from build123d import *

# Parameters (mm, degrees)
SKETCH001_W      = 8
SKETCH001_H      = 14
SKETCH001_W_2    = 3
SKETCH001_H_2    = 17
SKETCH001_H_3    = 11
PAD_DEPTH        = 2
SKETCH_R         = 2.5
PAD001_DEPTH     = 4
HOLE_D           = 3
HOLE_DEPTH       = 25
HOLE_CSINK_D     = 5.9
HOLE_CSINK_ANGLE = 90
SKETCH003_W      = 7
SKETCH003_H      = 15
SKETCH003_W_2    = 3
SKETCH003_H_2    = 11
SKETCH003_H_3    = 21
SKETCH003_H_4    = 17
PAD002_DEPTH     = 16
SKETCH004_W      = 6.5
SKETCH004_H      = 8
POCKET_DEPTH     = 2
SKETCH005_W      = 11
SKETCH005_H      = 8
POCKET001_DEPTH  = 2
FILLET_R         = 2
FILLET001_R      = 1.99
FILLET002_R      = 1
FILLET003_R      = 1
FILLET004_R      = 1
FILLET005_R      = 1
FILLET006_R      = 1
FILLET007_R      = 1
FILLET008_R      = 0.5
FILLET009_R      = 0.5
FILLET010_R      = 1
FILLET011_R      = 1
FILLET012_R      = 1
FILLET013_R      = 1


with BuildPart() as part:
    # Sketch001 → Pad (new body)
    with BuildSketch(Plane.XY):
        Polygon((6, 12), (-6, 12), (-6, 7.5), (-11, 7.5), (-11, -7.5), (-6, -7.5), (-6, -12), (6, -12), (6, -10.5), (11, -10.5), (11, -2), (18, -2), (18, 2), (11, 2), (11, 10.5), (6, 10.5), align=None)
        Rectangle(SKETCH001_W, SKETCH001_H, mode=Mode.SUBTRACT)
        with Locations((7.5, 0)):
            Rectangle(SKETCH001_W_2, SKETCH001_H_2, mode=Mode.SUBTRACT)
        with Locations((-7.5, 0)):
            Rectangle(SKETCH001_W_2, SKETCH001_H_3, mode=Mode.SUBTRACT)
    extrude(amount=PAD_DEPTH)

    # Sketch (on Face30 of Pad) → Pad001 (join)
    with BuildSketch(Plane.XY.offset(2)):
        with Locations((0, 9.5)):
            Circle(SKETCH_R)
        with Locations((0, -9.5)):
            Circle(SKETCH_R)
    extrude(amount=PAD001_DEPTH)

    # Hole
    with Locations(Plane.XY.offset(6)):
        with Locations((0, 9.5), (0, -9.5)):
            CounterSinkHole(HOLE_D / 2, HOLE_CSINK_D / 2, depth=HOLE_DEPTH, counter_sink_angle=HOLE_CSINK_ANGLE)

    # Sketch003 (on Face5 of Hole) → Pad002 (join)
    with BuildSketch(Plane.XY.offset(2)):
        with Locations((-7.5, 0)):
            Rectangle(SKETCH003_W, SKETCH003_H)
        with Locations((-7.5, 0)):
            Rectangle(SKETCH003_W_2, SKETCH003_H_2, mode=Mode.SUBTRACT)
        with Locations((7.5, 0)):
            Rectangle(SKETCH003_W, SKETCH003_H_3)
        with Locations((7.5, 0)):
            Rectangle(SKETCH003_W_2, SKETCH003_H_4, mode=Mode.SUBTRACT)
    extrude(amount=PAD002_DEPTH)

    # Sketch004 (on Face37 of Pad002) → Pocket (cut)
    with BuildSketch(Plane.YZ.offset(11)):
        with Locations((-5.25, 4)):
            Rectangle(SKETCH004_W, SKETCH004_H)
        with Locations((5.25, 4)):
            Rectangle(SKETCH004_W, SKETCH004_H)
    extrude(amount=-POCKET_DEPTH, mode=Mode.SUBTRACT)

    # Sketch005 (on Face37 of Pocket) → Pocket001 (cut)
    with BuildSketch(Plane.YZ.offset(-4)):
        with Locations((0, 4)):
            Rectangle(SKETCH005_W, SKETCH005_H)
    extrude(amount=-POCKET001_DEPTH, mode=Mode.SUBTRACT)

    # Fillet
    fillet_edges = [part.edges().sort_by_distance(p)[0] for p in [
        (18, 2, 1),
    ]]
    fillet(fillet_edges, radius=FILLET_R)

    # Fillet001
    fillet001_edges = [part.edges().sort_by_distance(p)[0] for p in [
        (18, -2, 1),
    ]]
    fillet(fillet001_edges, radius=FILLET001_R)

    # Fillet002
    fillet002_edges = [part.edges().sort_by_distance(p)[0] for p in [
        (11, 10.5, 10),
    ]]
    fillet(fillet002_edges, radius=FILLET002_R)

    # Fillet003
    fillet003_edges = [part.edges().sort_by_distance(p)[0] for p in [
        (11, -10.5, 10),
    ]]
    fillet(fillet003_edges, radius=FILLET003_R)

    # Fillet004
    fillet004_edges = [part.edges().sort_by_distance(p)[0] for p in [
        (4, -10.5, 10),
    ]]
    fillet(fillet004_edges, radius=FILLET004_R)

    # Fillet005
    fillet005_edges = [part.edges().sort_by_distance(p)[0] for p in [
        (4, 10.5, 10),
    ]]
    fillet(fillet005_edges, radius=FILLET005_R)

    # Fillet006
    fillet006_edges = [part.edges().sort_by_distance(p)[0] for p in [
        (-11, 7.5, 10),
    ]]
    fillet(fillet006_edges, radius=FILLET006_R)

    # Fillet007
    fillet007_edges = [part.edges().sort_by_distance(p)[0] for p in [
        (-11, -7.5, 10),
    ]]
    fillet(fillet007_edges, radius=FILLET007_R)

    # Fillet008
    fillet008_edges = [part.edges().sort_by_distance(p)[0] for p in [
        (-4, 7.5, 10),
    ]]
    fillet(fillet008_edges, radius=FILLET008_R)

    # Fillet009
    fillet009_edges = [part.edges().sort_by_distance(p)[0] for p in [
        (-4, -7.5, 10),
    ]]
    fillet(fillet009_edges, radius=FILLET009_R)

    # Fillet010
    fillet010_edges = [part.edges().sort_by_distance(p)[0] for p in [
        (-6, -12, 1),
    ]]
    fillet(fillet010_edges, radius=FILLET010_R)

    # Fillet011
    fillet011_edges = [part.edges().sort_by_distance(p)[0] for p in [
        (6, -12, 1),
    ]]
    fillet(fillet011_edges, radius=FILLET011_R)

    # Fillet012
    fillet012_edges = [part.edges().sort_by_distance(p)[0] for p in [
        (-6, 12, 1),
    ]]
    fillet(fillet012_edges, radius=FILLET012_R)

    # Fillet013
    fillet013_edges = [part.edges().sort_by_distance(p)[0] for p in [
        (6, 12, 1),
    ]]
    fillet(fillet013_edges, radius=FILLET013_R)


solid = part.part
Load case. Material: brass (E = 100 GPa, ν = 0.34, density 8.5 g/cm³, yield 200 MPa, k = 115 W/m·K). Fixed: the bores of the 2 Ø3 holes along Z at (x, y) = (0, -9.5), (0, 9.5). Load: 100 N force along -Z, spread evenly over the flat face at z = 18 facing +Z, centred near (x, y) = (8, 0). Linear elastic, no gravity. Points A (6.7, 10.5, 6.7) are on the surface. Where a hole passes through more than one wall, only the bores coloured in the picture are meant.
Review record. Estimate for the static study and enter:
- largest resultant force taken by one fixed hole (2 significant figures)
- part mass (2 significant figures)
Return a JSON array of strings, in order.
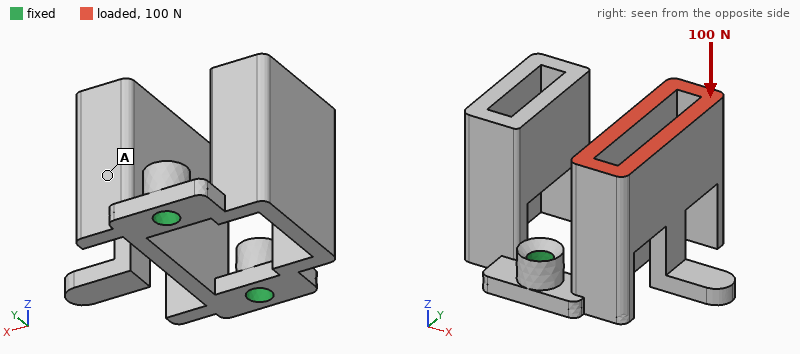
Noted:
["50 N", "25 g"]
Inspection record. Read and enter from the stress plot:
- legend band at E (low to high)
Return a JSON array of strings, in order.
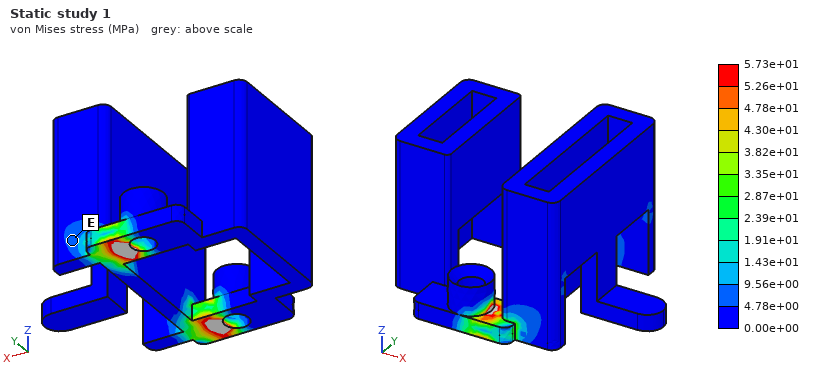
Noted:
["4.78e+00 to 9.56e+00 MPa"]
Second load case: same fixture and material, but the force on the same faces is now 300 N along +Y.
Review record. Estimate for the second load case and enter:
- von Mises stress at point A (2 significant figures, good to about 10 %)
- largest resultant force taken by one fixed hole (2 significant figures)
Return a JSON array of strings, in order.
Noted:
["16 MPa", "310 N"]
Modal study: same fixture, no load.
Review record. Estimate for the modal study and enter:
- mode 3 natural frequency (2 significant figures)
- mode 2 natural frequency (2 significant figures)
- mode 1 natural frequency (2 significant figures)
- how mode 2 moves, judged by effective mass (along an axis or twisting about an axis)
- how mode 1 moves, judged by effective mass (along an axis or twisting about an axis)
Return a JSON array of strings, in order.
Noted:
["4300 Hz", "1600 Hz", "1400 Hz", "along X", "along X"]
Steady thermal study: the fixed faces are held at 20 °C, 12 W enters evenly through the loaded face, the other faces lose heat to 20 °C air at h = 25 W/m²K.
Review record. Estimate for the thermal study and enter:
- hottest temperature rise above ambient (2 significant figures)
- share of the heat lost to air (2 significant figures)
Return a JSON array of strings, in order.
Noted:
["47 K", "13 %"]
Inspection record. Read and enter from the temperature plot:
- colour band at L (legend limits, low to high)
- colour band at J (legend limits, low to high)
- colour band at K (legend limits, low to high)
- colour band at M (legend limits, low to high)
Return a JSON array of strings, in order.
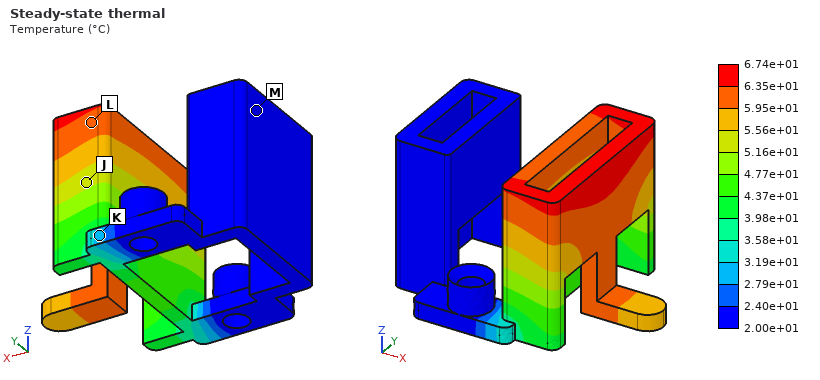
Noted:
["5.95e+01 to 6.35e+01 °C", "5.16e+01 to 5.56e+01 °C", "2.79e+01 to 3.19e+01 °C", "2.00e+01 to 2.40e+01 °C"]
